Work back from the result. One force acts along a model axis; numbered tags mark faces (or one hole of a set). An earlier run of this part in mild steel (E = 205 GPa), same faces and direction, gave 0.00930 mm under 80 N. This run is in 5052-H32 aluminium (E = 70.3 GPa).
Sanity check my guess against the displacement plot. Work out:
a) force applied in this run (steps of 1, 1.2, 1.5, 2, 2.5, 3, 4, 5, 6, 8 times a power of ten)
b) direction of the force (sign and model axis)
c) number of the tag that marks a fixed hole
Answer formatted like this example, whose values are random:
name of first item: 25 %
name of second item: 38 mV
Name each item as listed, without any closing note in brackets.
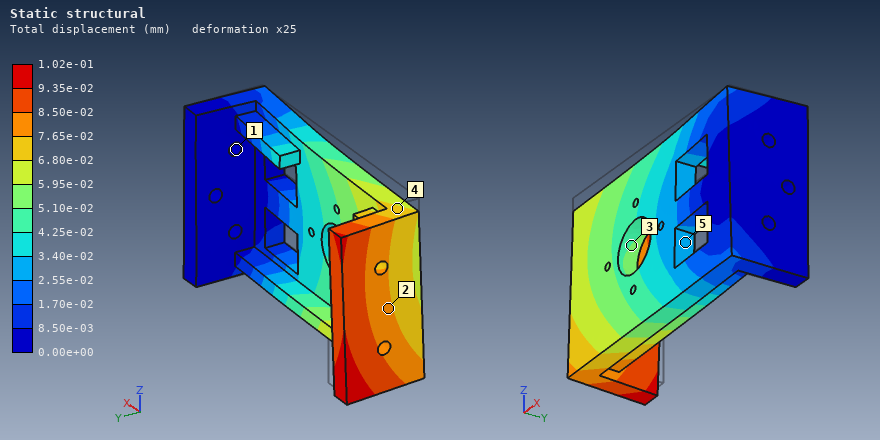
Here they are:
force applied in this run: 300 N
direction of the force: -Z
number of the tag that marks a fixed hole: 1
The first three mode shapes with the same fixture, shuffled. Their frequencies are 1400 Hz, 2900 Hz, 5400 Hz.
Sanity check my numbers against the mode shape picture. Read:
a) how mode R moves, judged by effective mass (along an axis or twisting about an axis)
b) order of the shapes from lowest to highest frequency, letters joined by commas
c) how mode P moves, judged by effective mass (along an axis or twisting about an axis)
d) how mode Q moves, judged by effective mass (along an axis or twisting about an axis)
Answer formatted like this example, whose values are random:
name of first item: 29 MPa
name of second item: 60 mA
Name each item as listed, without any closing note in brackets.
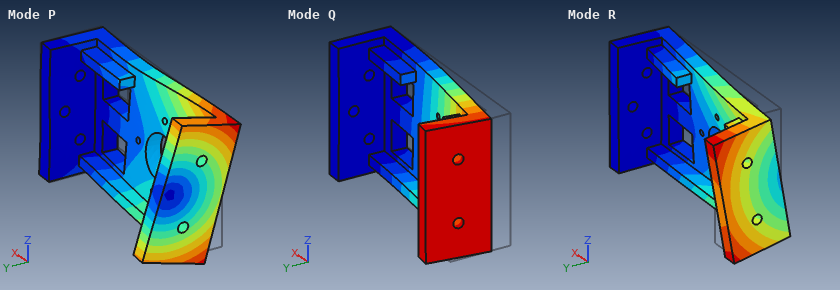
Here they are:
how mode R moves, judged by effective mass: along Z
order of the shapes from lowest to highest frequency, letters joined by commas: Q, R, P
how mode P moves, judged by effective mass: along Z
how mode Q moves, judged by effective mass: along Y
